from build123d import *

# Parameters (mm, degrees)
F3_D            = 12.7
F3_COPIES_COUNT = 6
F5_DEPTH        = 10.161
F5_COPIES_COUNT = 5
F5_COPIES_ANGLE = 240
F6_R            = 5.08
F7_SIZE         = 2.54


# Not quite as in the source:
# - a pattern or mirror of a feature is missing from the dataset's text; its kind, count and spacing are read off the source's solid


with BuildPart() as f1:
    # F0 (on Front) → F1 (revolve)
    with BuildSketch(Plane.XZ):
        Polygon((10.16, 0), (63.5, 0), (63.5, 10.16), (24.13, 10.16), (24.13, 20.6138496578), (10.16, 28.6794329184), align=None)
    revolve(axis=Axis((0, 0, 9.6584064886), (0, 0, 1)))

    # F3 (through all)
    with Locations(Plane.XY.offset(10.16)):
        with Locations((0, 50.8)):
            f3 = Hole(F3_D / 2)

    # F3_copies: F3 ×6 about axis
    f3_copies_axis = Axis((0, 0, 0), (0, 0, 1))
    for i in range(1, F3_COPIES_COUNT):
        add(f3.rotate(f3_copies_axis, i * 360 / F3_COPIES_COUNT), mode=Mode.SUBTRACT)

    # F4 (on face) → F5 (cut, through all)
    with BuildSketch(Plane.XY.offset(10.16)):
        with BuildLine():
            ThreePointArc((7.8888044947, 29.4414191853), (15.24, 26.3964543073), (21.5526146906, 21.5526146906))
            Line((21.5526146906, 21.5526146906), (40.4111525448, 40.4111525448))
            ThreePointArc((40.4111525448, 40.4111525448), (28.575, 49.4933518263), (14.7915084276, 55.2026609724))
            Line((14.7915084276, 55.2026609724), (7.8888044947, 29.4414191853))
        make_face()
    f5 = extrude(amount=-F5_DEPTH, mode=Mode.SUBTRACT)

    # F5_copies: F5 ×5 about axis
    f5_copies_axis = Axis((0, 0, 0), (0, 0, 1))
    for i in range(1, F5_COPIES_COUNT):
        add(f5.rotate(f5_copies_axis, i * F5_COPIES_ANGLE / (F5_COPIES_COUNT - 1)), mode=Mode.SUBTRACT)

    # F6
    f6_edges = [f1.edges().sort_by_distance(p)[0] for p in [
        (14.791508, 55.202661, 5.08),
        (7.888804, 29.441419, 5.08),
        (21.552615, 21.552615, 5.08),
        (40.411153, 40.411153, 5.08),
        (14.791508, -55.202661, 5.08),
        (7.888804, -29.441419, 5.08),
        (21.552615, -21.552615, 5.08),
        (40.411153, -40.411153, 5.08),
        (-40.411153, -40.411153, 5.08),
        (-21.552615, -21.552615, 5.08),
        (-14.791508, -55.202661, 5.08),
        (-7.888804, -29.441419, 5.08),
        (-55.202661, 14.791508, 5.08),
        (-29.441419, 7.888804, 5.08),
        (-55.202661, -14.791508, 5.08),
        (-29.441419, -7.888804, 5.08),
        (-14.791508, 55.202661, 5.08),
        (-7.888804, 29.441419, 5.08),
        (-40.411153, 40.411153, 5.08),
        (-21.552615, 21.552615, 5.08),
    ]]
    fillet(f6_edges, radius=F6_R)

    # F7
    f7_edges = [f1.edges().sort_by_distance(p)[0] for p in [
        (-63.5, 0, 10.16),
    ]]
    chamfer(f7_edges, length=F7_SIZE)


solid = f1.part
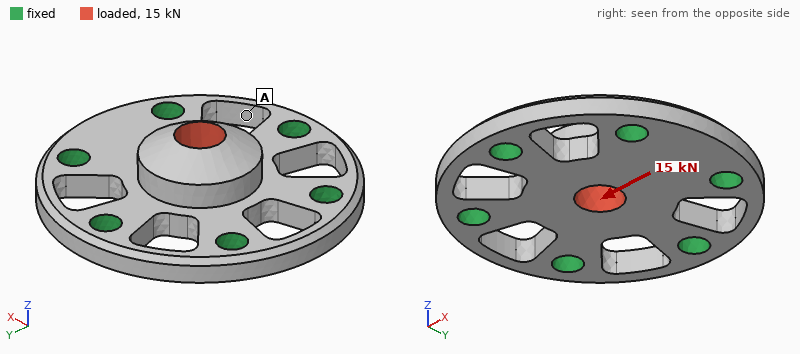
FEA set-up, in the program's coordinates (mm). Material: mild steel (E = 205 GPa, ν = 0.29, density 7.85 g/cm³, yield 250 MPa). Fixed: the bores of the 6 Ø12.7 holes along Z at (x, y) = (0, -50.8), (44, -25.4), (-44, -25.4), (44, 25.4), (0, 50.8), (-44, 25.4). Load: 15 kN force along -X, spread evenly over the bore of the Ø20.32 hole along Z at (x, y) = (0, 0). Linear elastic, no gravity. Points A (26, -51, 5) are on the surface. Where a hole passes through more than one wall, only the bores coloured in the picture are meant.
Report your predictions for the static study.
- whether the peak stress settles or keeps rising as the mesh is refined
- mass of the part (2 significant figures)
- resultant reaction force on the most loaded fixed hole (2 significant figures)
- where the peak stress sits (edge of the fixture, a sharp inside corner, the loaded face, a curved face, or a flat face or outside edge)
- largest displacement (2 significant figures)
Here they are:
keeps rising
840 g
3.9 kN
edge of the fixture
9.0 µm
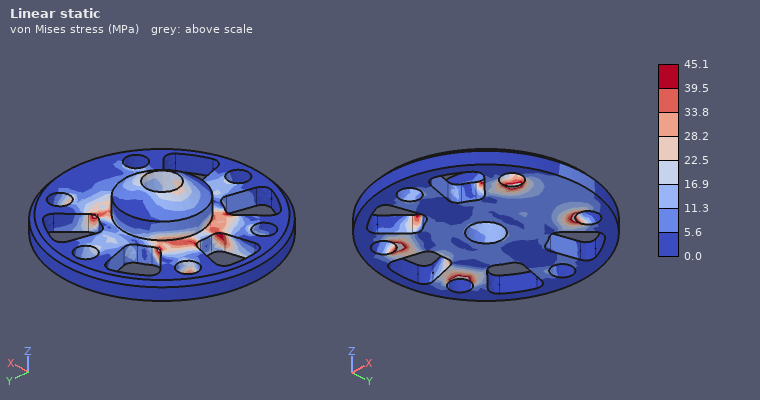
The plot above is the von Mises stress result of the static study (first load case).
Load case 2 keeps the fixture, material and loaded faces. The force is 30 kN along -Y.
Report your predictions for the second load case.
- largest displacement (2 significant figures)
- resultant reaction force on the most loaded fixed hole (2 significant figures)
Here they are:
19 µm
8.3 kN
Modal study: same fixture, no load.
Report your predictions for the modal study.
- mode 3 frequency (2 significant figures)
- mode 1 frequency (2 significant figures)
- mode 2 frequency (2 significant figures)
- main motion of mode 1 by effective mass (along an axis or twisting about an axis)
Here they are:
13 kHz
8500 Hz
13 kHz
along Z
